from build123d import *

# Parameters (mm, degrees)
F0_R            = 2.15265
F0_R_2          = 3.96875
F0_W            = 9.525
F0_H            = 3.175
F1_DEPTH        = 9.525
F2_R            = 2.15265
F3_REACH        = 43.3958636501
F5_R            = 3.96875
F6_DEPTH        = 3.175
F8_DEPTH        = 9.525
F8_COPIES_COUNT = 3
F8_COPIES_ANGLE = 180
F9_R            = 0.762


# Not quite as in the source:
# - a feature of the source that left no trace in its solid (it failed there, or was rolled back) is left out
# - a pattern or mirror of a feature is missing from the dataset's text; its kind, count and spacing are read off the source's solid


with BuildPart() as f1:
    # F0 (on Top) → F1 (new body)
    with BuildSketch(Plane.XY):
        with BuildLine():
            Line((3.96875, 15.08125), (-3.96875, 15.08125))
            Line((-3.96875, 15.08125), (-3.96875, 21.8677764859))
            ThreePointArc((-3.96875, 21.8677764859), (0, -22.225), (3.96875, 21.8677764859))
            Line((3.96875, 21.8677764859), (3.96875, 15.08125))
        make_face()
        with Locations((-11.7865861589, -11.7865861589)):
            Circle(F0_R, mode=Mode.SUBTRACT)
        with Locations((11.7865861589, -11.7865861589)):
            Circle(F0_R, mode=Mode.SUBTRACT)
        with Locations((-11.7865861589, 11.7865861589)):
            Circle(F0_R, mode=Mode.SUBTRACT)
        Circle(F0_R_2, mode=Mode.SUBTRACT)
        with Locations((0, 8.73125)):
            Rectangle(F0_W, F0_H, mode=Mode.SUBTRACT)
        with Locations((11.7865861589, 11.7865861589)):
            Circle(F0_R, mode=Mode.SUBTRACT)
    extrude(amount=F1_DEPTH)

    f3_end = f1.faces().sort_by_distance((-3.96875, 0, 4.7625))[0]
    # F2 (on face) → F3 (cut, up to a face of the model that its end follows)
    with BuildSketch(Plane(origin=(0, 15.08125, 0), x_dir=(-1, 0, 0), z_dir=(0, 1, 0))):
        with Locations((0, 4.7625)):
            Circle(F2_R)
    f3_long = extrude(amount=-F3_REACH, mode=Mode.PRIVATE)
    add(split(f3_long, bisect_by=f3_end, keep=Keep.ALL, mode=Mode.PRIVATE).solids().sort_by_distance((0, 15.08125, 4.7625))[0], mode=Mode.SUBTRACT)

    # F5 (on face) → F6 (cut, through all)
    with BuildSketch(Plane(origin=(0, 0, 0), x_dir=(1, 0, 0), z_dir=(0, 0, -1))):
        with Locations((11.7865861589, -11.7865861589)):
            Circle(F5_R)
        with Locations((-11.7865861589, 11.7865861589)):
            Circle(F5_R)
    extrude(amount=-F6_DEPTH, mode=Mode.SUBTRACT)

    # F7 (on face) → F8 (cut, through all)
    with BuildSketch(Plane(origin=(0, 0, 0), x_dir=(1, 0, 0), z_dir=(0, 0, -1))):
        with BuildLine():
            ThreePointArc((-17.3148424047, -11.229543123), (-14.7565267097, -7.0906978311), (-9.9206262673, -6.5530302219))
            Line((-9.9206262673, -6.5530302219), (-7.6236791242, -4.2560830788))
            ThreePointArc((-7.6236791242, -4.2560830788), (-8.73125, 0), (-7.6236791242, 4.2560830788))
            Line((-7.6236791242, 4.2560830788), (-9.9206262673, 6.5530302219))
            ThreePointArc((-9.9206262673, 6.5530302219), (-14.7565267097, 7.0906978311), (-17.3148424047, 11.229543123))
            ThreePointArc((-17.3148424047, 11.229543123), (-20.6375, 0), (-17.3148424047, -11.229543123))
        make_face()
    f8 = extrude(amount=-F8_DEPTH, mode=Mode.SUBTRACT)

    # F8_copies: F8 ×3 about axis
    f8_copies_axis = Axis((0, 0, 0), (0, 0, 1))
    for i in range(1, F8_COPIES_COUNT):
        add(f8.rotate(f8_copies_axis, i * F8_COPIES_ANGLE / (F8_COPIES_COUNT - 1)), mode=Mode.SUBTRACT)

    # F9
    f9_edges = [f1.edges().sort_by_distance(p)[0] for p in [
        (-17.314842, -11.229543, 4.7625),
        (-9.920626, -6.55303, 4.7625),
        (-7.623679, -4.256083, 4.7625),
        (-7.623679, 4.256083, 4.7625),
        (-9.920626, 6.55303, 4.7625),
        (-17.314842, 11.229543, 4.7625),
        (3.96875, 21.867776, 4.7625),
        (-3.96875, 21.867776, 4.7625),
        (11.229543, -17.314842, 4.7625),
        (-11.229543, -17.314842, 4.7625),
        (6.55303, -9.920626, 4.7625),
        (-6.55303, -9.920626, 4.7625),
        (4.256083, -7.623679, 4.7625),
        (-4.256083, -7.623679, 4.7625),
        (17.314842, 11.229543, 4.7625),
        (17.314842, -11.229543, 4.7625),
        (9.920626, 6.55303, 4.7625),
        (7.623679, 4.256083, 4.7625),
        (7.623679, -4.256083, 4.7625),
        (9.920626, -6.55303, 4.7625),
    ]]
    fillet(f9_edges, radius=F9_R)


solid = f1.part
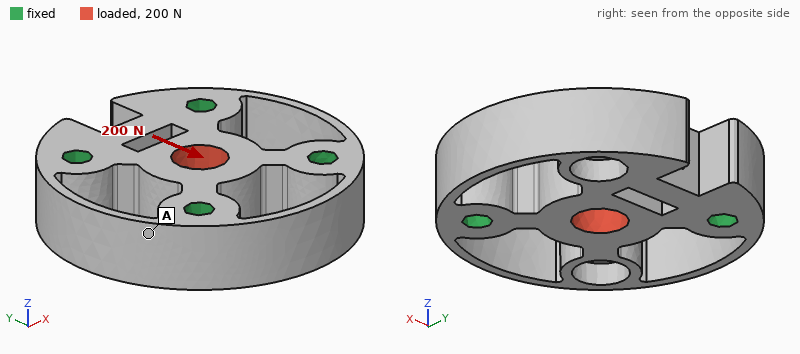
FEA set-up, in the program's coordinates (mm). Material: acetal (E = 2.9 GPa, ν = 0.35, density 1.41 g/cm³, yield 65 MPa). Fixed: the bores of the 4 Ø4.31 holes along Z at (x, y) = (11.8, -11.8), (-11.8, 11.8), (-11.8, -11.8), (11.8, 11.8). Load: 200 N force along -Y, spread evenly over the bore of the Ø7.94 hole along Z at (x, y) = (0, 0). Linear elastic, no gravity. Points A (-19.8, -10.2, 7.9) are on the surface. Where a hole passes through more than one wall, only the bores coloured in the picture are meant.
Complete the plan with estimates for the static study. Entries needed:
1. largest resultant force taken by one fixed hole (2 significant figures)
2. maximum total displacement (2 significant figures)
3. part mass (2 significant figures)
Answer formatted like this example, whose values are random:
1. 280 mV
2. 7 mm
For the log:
1. 61 N
2. 8.9 µm
3. 11 g
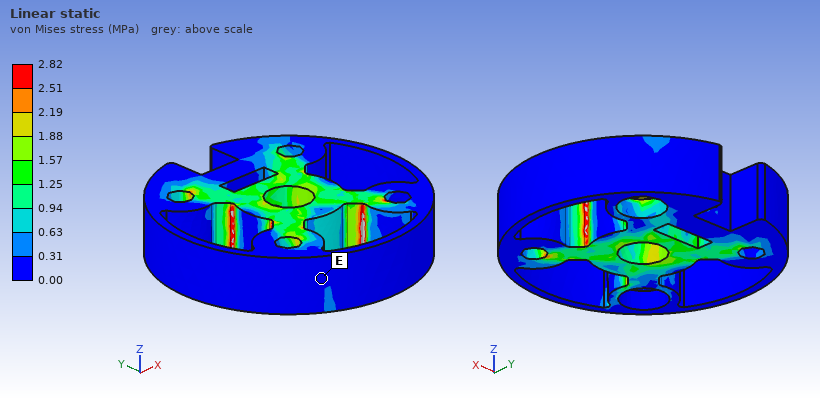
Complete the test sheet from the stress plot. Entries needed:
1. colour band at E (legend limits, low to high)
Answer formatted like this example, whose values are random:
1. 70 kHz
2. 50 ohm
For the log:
1. 0.00 to 0.31 MPa
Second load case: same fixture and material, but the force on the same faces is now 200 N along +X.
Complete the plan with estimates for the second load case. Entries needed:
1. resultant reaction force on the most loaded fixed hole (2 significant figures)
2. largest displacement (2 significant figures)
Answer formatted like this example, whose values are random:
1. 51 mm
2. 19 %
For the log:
1. 68 N
2. 9.8 µm
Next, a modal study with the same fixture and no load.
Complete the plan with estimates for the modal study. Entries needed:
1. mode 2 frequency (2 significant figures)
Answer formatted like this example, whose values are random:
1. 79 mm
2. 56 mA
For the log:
1. 8200 Hz
